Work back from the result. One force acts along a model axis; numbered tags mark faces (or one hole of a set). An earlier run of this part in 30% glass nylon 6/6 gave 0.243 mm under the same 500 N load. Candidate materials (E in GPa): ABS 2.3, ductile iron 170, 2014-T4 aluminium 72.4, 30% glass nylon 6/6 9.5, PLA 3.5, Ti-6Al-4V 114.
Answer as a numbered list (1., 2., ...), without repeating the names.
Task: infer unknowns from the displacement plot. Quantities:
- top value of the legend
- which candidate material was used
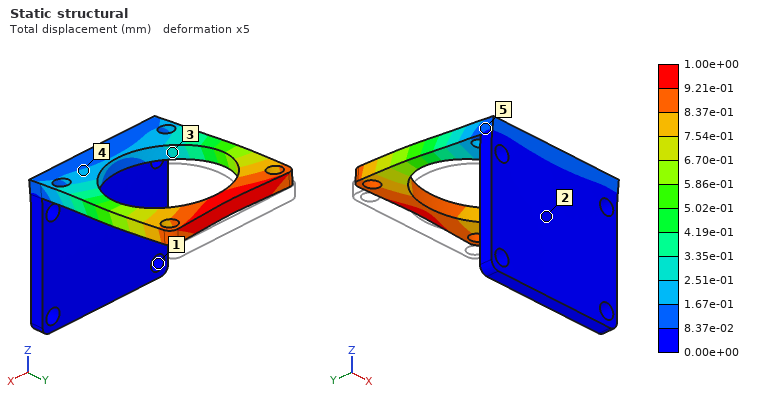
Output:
1. 1.00e+00 mm
2. ABS
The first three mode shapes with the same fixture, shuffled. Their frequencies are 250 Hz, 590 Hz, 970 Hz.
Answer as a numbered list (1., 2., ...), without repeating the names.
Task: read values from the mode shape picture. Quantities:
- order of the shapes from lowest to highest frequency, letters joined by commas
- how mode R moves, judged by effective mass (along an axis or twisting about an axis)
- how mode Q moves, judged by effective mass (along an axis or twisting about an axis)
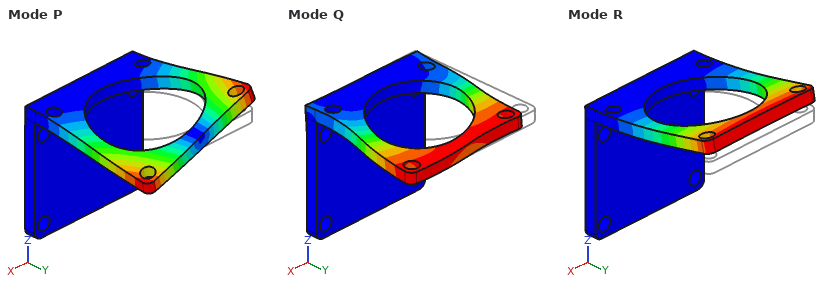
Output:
1. R, P, Q
2. along Z
3. along X
